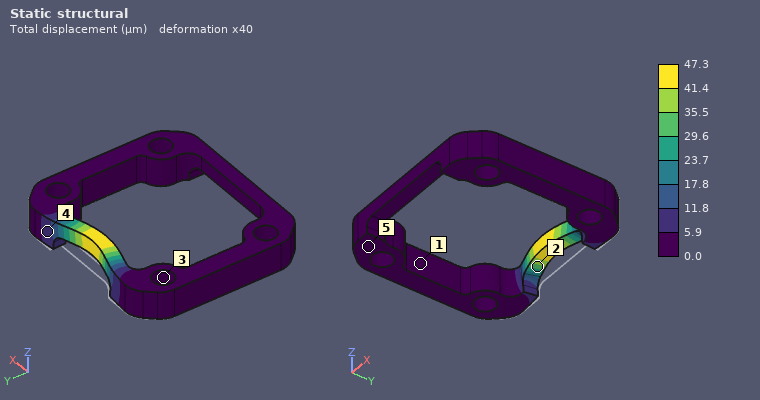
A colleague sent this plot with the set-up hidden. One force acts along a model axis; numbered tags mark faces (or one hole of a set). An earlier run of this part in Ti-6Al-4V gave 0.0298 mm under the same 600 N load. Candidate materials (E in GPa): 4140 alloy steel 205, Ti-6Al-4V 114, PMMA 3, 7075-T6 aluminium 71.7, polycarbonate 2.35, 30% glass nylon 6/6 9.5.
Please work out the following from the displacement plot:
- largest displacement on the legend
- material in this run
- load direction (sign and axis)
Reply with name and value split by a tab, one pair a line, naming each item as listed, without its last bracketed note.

largest displacement on the legend	47.3 µm
material in this run	7075-T6 aluminium
load direction	-Y
